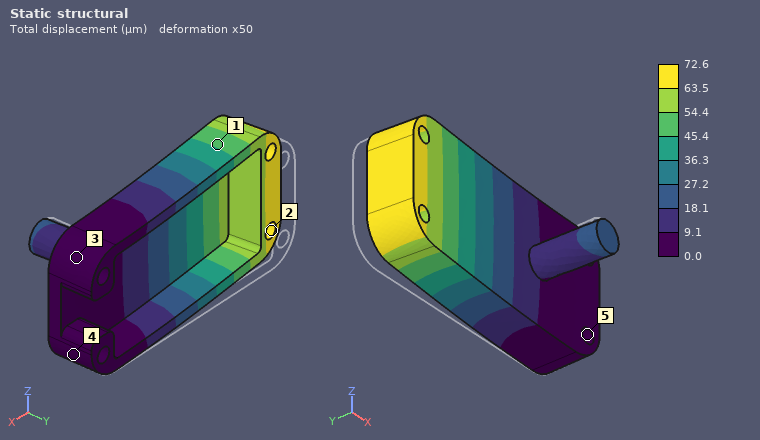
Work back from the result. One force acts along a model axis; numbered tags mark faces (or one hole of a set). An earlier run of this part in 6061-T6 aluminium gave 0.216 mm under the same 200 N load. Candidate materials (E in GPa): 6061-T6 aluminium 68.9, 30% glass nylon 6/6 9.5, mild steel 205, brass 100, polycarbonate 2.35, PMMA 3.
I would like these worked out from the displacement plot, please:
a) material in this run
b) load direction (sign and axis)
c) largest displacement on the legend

mild steel
-Y
72.6 µm
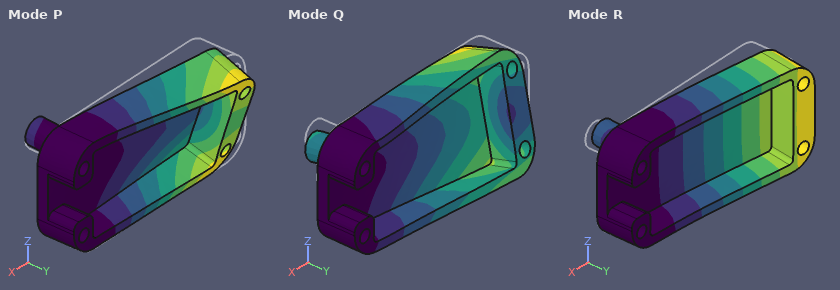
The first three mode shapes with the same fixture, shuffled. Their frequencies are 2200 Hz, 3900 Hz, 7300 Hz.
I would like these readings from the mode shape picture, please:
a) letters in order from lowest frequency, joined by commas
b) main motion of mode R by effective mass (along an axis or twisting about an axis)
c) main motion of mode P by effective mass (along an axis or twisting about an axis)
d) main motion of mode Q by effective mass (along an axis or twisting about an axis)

R, P, Q
along Y
along Z
along Z
